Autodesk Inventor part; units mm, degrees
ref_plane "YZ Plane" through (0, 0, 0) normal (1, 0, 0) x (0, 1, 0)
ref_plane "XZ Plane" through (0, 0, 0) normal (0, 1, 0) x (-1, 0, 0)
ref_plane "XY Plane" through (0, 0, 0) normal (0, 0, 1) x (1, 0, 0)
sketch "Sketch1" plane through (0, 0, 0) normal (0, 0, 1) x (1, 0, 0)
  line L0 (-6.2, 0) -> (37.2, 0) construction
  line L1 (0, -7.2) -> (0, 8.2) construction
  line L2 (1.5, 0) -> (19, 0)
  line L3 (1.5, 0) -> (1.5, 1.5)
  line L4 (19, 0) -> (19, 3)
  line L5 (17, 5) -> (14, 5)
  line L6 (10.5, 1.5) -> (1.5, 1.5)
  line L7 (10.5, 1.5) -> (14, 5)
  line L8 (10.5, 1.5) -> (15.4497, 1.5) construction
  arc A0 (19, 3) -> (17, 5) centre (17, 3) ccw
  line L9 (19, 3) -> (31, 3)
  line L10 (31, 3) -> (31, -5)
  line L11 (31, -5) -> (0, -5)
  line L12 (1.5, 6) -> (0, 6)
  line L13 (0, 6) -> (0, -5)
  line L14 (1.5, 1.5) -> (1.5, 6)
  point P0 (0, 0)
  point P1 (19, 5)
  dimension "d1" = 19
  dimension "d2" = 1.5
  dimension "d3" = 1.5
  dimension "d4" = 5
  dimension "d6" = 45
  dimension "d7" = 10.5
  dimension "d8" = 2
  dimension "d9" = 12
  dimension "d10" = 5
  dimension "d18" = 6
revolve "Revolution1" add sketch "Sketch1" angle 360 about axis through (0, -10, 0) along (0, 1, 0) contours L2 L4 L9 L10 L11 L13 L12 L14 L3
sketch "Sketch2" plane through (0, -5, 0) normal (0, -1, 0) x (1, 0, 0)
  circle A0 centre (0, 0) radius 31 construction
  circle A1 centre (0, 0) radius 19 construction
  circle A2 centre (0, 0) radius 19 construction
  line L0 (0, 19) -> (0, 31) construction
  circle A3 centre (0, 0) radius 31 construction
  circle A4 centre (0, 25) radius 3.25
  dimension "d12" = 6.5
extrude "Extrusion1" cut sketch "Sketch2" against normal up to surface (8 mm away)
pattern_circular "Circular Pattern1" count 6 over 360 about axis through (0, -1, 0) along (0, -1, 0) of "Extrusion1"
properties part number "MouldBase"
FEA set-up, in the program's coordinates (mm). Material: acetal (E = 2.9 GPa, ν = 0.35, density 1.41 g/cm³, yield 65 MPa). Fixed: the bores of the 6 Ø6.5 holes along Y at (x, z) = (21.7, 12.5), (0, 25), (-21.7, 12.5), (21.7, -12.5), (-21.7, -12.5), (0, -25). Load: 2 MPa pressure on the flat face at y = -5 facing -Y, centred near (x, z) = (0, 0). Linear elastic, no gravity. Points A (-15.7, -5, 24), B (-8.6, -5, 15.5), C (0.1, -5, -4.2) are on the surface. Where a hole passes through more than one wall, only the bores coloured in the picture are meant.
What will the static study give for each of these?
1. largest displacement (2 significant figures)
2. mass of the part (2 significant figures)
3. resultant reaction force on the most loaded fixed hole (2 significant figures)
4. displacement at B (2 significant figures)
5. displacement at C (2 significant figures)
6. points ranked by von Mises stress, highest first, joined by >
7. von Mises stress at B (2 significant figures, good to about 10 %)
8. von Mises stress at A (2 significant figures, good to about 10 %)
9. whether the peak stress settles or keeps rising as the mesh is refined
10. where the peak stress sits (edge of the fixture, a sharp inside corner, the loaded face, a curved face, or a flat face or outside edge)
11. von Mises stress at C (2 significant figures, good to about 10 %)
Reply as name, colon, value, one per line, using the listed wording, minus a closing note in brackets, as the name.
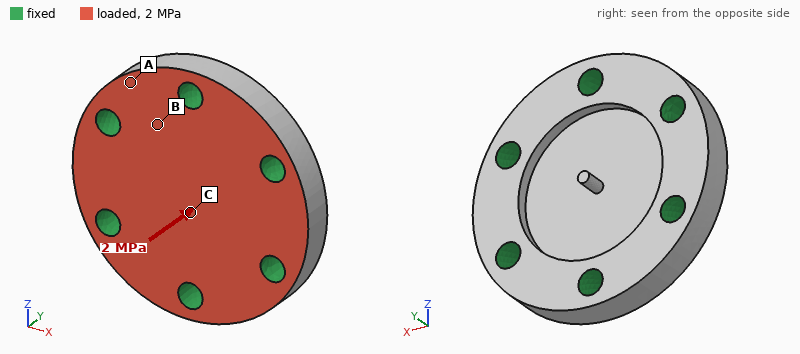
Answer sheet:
largest displacement: 0.26 mm
mass of the part: 27 g
resultant reaction force on the most loaded fixed hole: 950 N
displacement at B: 0.073 mm
displacement at C: 0.25 mm
points ranked by von Mises stress, highest first, joined by >: C > B > A
von Mises stress at B: 12 MPa
von Mises stress at A: 3.9 MPa
whether the peak stress settles or keeps rising as the mesh is refined: keeps rising
where the peak stress sits: edge of the fixture
von Mises stress at C: 18 MPa
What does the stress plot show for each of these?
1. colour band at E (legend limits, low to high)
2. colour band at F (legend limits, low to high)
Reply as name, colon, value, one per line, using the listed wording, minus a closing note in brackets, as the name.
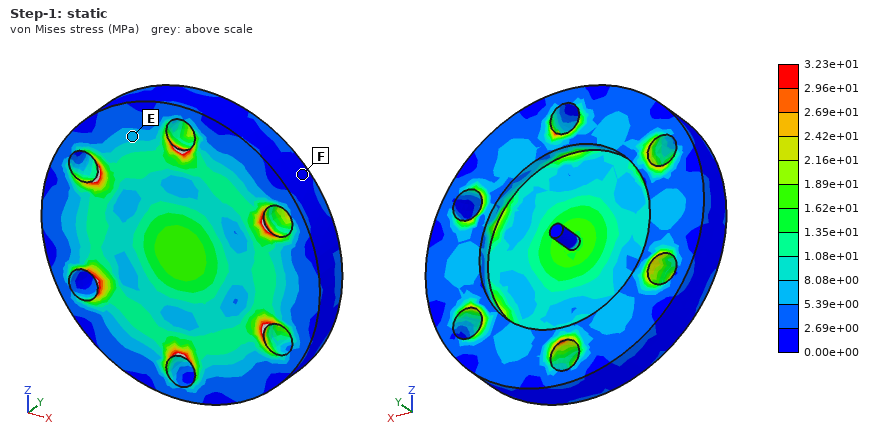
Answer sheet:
colour band at E: 5.39e+00 to 8.08e+00 MPa
colour band at F: 0.00e+00 to 2.69e+00 MPa
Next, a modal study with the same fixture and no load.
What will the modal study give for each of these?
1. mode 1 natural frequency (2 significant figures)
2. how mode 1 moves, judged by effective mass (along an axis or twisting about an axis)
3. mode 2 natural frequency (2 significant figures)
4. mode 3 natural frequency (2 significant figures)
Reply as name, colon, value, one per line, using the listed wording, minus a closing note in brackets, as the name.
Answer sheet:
mode 1 natural frequency: 6300 Hz
how mode 1 moves, judged by effective mass: along Y
mode 2 natural frequency: 11 kHz
mode 3 natural frequency: 11 kHz
